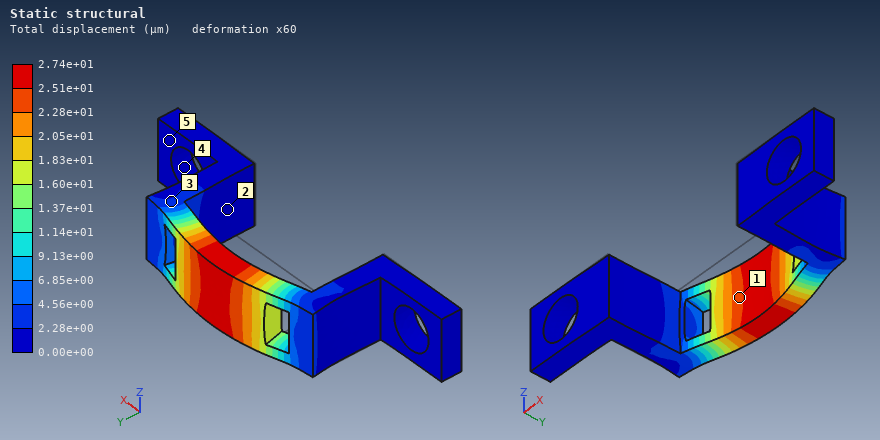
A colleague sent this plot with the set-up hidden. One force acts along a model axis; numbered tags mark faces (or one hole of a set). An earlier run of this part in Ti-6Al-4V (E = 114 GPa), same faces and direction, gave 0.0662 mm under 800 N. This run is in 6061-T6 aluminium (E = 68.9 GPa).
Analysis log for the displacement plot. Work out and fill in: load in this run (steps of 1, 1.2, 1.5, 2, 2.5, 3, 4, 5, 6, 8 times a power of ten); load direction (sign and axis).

200 N
+Y
